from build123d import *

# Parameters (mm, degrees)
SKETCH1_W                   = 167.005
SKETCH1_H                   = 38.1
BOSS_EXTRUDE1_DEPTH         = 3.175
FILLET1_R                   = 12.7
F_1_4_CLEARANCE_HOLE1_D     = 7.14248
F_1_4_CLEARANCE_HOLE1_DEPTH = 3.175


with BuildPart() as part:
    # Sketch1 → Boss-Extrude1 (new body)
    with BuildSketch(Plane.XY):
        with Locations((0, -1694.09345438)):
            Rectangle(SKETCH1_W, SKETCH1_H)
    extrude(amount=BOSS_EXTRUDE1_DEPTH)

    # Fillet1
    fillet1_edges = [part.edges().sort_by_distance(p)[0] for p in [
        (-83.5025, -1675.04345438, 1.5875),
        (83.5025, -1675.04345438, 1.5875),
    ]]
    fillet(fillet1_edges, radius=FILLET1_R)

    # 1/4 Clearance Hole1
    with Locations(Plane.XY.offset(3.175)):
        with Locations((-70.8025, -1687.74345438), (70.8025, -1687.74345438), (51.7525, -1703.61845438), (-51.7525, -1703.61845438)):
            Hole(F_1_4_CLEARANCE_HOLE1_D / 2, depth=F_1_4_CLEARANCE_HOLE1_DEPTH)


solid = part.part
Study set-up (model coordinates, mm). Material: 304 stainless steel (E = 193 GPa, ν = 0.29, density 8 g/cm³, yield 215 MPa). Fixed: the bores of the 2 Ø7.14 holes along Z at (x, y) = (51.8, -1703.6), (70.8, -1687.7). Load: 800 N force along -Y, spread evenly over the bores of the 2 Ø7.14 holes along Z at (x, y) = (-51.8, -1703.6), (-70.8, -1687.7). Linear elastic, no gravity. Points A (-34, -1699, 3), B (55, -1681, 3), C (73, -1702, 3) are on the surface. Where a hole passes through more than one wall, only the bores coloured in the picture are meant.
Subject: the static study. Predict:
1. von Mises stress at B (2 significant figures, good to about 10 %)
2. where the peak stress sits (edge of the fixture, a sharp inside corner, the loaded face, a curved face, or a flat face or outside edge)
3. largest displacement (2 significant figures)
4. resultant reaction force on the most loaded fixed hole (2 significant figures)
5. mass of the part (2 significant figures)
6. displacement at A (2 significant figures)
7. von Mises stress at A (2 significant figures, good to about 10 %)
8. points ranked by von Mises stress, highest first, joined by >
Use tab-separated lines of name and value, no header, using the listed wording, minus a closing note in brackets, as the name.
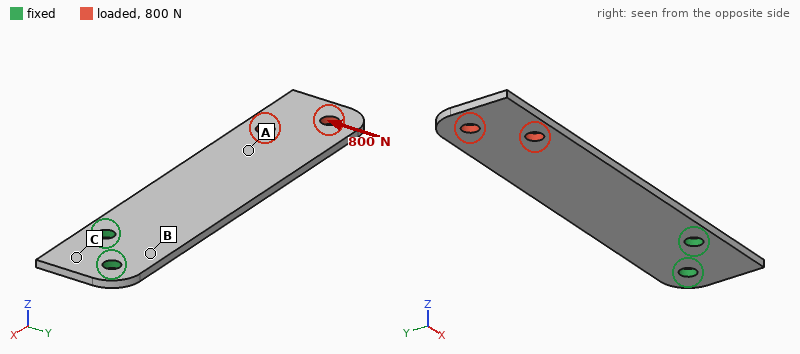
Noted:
von Mises stress at B	71 MPa
where the peak stress sits	edge of the fixture
largest displacement	0.23 mm
resultant reaction force on the most loaded fixed hole	3.6 kN
mass of the part	160 g
displacement at A	0.12 mm
von Mises stress at A	18 MPa
points ranked by von Mises stress, highest first, joined by >	B > A > C
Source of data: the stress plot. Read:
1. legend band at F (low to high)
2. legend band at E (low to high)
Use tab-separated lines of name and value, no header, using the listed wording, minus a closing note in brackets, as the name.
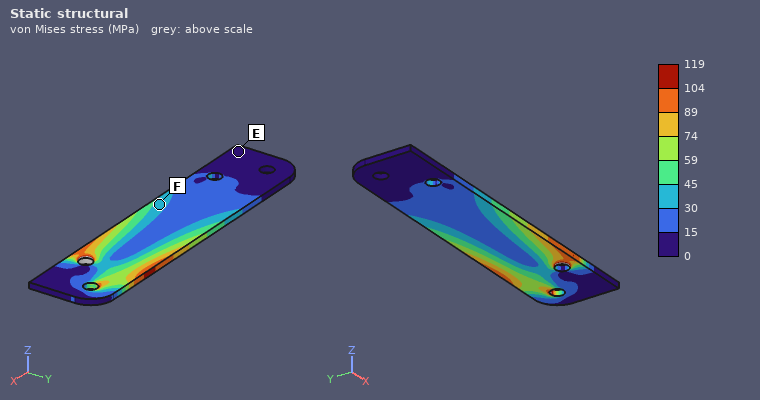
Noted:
legend band at F	30 to 45 MPa
legend band at E	0 to 15 MPa
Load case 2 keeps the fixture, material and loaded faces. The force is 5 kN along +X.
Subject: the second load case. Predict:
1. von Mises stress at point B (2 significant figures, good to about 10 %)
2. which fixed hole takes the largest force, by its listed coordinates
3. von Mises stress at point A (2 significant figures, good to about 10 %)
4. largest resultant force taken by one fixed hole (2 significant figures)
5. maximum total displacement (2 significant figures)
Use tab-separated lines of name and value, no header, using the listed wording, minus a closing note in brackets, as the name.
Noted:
von Mises stress at point B	34 MPa
which fixed hole takes the largest force, by its listed coordinates	(51.8, -1703.6)
von Mises stress at point A	45 MPa
largest resultant force taken by one fixed hole	3.1 kN
maximum total displacement	28 µm
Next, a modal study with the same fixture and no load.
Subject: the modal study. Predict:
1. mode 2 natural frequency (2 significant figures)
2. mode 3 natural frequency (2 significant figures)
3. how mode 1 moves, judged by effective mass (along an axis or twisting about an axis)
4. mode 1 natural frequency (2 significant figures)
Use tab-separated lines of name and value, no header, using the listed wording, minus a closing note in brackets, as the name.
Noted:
mode 2 natural frequency	840 Hz
mode 3 natural frequency	990 Hz
how mode 1 moves, judged by effective mass	along Z
mode 1 natural frequency	140 Hz
